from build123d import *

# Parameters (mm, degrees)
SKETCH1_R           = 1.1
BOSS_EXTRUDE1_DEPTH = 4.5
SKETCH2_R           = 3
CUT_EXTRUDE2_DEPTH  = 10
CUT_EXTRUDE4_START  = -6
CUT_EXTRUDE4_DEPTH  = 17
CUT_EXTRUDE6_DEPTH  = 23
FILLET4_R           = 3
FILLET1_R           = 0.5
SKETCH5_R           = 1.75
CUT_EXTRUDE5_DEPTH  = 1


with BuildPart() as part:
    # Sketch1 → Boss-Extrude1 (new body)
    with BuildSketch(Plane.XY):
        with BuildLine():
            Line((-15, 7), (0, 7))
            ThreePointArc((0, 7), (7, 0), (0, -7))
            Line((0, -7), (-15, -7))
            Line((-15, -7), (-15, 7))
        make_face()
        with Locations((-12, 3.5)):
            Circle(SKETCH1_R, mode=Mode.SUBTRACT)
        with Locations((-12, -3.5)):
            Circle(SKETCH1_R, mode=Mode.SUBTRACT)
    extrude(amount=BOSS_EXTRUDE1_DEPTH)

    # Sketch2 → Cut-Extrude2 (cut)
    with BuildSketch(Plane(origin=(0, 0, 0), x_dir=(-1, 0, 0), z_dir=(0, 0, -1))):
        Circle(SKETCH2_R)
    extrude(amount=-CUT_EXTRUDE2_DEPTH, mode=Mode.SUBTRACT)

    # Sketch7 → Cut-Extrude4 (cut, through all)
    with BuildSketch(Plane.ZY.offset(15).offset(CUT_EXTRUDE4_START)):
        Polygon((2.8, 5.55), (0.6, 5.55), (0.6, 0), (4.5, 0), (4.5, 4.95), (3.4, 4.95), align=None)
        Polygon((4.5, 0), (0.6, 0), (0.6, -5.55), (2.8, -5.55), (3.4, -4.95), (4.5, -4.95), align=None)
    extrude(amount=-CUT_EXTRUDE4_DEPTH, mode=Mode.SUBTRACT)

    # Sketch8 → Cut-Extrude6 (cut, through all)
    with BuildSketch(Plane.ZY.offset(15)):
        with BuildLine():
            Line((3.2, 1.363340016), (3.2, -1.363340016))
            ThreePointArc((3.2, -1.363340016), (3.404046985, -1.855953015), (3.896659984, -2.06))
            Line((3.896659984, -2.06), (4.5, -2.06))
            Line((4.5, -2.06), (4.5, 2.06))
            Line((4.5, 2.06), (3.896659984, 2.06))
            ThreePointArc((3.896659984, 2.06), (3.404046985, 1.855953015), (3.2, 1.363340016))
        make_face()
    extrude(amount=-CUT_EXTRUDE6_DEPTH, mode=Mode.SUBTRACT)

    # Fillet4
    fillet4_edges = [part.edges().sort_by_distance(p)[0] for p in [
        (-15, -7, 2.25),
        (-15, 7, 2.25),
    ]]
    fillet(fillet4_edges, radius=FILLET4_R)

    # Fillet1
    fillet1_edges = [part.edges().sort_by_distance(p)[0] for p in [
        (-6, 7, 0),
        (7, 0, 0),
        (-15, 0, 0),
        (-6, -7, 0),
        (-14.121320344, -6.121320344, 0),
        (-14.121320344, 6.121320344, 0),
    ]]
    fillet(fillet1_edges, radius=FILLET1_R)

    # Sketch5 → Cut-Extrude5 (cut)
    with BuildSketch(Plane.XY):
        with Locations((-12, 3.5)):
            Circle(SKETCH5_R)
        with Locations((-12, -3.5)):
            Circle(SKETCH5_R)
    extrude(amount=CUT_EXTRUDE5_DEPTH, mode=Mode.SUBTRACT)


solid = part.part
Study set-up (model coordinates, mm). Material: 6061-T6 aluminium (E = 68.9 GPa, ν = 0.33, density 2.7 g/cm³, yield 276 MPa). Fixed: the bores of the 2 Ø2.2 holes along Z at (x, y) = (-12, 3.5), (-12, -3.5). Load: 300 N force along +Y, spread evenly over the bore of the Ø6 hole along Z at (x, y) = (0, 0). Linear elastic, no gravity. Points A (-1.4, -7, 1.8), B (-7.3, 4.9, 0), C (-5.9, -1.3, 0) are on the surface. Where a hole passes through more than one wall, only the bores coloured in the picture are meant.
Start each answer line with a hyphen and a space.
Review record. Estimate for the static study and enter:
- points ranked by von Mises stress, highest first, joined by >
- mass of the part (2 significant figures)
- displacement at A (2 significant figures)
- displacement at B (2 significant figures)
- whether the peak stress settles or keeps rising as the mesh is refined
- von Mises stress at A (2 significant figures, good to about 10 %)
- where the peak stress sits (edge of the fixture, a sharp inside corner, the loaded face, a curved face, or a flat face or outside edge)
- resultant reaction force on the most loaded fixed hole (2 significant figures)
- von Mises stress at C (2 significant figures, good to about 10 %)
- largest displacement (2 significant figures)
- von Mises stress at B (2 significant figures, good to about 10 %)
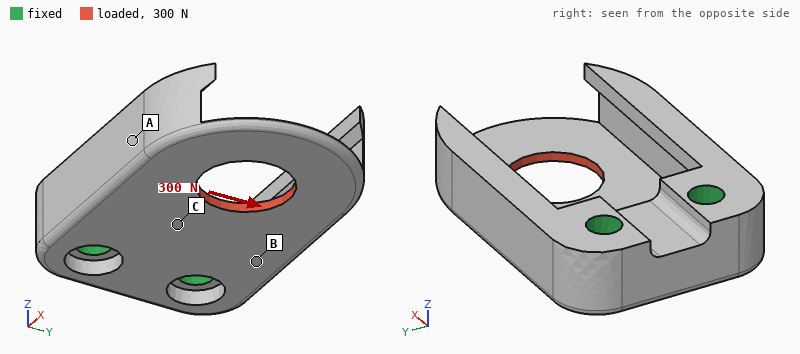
- C > B > A
- 1.5 g
- 31 µm
- 9.2 µm
- keeps rising
- 20 MPa
- a sharp inside corner
- 380 N
- 83 MPa
- 59 µm
- 55 MPa
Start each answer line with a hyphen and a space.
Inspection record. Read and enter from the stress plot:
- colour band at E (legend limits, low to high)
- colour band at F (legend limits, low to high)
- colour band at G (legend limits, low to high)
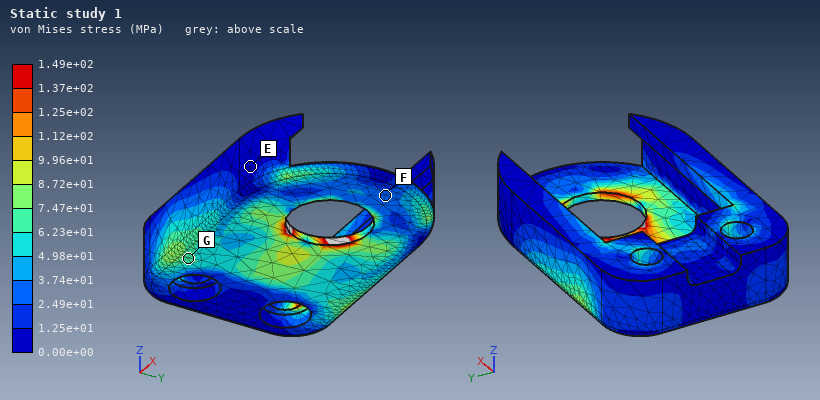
- 0.00e+00 to 1.25e+01 MPa
- 2.49e+01 to 3.74e+01 MPa
- 6.23e+01 to 7.47e+01 MPa
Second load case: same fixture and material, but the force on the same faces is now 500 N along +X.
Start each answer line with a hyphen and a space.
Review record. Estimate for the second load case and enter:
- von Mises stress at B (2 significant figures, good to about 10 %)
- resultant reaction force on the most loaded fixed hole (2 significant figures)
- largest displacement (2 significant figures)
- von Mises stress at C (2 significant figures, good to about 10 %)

- 51 MPa
- 250 N
- 43 µm
- 57 MPa
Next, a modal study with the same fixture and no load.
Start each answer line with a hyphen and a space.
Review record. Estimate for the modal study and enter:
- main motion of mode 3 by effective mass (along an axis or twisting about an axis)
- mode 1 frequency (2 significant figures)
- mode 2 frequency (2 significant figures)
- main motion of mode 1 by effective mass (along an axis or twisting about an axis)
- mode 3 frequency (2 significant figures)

- along Y
- 11 kHz
- 15 kHz
- along Z
- 20 kHz
